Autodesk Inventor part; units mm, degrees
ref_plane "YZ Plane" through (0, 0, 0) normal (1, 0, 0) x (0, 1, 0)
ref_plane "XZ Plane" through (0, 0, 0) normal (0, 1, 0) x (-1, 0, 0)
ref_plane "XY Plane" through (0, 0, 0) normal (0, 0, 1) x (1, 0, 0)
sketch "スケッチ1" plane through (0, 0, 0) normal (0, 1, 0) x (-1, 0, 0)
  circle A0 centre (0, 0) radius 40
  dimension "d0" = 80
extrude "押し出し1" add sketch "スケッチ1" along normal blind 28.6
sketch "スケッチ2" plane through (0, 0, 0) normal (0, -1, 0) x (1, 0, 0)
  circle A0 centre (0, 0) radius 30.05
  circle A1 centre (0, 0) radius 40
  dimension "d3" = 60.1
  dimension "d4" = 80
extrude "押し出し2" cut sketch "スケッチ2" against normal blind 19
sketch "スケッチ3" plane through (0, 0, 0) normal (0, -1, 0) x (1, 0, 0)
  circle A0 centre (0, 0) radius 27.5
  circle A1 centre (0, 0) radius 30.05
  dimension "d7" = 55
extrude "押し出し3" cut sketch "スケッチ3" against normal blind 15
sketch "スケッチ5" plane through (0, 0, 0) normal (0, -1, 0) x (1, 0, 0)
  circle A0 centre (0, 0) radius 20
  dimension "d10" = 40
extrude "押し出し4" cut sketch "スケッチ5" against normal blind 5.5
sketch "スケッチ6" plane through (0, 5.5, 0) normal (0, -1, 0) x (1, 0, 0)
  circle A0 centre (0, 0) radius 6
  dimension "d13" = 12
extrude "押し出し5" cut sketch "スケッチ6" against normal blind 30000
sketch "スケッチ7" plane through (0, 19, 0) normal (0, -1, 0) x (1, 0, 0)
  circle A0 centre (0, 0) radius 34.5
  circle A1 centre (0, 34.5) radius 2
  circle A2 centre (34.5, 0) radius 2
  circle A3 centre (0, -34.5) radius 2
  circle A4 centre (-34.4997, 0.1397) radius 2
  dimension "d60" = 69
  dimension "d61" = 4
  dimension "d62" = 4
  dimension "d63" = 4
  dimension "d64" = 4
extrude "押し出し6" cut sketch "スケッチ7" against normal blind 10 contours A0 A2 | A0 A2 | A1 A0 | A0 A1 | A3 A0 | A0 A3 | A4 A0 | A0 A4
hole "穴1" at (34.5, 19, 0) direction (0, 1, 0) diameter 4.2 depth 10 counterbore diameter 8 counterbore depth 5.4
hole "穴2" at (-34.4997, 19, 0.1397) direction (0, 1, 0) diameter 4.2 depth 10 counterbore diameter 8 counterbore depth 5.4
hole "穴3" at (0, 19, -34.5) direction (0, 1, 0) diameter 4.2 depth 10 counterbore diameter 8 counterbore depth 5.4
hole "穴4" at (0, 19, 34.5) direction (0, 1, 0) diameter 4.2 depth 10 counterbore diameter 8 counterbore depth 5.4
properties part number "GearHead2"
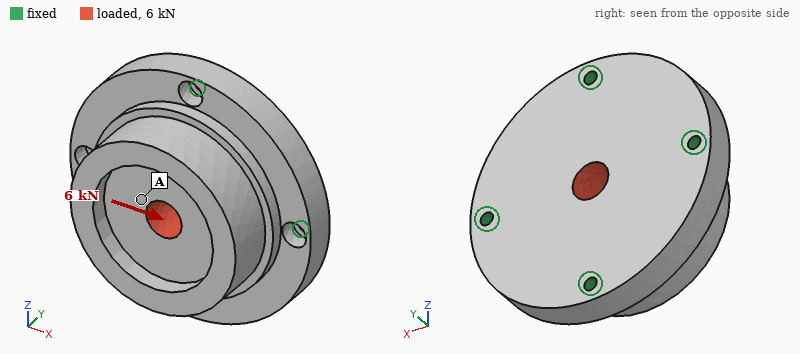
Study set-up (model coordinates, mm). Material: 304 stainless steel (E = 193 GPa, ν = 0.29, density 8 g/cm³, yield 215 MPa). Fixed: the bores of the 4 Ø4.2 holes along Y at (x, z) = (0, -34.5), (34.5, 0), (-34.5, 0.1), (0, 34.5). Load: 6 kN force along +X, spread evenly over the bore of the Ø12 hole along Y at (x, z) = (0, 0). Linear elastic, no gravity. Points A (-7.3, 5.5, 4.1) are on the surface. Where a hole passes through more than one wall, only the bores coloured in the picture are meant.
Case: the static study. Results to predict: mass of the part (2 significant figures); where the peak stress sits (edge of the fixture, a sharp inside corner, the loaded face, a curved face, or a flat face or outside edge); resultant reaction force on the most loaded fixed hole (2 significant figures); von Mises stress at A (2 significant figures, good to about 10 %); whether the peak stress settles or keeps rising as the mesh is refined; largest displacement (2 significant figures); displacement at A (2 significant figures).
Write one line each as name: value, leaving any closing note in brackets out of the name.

mass of the part: 680 g
where the peak stress sits: edge of the fixture
resultant reaction force on the most loaded fixed hole: 2.0 kN
von Mises stress at A: 7.4 MPa
whether the peak stress settles or keeps rising as the mesh is refined: keeps rising
largest displacement: 2.5 µm
displacement at A: 2.4 µm
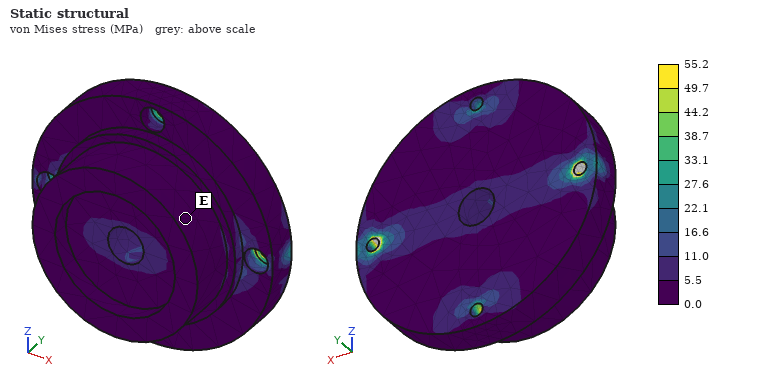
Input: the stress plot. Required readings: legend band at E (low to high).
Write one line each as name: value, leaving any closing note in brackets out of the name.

legend band at E: 0.0 to 5.5 MPa
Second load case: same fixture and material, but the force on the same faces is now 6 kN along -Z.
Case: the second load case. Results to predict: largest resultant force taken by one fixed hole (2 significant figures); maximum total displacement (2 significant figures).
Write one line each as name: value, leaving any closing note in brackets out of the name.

largest resultant force taken by one fixed hole: 2.0 kN
maximum total displacement: 2.5 µm
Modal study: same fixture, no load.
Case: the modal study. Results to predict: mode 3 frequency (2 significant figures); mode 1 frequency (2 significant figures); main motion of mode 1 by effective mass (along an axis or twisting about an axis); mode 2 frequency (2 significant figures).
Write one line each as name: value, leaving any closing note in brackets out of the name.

mode 3 frequency: 10 kHz
mode 1 frequency: 9400 Hz
main motion of mode 1 by effective mass: along Y
mode 2 frequency: 10 kHz
